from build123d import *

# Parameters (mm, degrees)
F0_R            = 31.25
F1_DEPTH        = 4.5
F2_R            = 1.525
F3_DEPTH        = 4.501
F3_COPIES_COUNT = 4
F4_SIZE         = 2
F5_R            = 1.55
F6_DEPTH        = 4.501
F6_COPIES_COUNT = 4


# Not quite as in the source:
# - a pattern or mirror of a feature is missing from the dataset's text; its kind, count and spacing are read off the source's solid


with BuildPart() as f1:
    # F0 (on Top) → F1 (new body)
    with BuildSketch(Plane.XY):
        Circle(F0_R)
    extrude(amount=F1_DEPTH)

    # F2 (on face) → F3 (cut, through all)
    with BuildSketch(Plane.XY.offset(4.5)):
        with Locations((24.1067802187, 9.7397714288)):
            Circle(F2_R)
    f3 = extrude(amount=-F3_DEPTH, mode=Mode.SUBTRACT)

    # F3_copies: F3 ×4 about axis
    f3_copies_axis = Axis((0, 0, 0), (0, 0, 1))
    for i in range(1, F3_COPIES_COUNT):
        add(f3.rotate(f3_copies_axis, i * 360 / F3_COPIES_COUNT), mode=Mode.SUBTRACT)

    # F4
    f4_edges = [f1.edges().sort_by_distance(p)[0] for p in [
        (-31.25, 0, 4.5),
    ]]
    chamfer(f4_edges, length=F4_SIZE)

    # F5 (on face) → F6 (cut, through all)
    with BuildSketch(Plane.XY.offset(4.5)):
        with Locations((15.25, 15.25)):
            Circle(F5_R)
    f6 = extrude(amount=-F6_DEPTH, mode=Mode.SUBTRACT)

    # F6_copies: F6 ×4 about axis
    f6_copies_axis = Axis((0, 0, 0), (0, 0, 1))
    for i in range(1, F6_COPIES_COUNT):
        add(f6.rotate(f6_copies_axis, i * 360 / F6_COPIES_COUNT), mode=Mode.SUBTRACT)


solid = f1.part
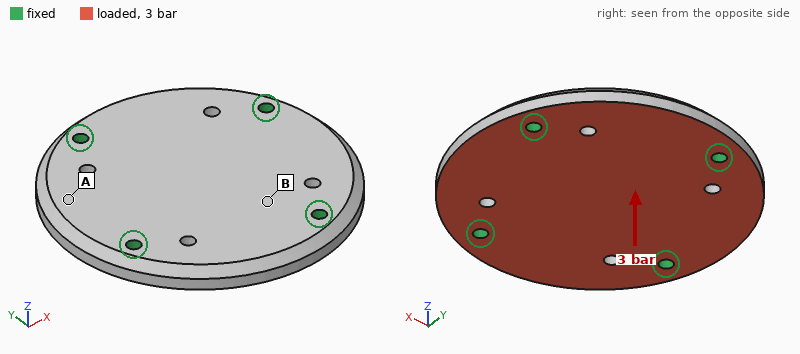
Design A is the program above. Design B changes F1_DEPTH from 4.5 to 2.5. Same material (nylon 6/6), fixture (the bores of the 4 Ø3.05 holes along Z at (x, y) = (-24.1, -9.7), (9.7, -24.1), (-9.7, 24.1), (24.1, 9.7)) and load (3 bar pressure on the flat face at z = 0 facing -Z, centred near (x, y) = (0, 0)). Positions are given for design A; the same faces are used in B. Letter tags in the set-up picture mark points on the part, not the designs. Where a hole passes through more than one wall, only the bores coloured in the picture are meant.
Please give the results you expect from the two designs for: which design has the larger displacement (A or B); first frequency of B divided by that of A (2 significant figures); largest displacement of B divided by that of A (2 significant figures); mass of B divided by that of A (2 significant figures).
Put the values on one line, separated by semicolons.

B; 0.62; 4.7; 0.54
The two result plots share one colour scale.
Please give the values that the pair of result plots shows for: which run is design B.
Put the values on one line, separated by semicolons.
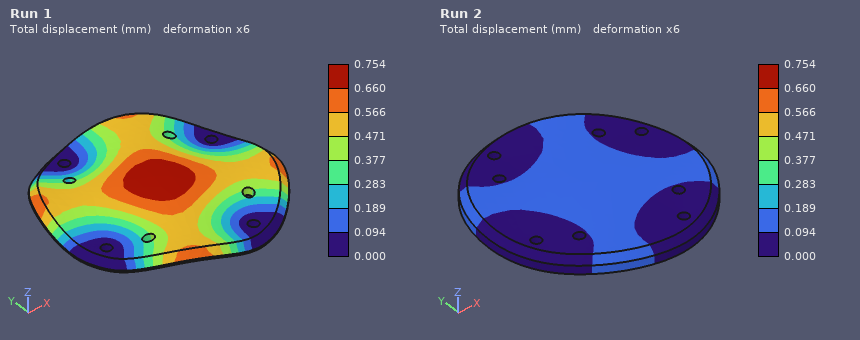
Run 1
